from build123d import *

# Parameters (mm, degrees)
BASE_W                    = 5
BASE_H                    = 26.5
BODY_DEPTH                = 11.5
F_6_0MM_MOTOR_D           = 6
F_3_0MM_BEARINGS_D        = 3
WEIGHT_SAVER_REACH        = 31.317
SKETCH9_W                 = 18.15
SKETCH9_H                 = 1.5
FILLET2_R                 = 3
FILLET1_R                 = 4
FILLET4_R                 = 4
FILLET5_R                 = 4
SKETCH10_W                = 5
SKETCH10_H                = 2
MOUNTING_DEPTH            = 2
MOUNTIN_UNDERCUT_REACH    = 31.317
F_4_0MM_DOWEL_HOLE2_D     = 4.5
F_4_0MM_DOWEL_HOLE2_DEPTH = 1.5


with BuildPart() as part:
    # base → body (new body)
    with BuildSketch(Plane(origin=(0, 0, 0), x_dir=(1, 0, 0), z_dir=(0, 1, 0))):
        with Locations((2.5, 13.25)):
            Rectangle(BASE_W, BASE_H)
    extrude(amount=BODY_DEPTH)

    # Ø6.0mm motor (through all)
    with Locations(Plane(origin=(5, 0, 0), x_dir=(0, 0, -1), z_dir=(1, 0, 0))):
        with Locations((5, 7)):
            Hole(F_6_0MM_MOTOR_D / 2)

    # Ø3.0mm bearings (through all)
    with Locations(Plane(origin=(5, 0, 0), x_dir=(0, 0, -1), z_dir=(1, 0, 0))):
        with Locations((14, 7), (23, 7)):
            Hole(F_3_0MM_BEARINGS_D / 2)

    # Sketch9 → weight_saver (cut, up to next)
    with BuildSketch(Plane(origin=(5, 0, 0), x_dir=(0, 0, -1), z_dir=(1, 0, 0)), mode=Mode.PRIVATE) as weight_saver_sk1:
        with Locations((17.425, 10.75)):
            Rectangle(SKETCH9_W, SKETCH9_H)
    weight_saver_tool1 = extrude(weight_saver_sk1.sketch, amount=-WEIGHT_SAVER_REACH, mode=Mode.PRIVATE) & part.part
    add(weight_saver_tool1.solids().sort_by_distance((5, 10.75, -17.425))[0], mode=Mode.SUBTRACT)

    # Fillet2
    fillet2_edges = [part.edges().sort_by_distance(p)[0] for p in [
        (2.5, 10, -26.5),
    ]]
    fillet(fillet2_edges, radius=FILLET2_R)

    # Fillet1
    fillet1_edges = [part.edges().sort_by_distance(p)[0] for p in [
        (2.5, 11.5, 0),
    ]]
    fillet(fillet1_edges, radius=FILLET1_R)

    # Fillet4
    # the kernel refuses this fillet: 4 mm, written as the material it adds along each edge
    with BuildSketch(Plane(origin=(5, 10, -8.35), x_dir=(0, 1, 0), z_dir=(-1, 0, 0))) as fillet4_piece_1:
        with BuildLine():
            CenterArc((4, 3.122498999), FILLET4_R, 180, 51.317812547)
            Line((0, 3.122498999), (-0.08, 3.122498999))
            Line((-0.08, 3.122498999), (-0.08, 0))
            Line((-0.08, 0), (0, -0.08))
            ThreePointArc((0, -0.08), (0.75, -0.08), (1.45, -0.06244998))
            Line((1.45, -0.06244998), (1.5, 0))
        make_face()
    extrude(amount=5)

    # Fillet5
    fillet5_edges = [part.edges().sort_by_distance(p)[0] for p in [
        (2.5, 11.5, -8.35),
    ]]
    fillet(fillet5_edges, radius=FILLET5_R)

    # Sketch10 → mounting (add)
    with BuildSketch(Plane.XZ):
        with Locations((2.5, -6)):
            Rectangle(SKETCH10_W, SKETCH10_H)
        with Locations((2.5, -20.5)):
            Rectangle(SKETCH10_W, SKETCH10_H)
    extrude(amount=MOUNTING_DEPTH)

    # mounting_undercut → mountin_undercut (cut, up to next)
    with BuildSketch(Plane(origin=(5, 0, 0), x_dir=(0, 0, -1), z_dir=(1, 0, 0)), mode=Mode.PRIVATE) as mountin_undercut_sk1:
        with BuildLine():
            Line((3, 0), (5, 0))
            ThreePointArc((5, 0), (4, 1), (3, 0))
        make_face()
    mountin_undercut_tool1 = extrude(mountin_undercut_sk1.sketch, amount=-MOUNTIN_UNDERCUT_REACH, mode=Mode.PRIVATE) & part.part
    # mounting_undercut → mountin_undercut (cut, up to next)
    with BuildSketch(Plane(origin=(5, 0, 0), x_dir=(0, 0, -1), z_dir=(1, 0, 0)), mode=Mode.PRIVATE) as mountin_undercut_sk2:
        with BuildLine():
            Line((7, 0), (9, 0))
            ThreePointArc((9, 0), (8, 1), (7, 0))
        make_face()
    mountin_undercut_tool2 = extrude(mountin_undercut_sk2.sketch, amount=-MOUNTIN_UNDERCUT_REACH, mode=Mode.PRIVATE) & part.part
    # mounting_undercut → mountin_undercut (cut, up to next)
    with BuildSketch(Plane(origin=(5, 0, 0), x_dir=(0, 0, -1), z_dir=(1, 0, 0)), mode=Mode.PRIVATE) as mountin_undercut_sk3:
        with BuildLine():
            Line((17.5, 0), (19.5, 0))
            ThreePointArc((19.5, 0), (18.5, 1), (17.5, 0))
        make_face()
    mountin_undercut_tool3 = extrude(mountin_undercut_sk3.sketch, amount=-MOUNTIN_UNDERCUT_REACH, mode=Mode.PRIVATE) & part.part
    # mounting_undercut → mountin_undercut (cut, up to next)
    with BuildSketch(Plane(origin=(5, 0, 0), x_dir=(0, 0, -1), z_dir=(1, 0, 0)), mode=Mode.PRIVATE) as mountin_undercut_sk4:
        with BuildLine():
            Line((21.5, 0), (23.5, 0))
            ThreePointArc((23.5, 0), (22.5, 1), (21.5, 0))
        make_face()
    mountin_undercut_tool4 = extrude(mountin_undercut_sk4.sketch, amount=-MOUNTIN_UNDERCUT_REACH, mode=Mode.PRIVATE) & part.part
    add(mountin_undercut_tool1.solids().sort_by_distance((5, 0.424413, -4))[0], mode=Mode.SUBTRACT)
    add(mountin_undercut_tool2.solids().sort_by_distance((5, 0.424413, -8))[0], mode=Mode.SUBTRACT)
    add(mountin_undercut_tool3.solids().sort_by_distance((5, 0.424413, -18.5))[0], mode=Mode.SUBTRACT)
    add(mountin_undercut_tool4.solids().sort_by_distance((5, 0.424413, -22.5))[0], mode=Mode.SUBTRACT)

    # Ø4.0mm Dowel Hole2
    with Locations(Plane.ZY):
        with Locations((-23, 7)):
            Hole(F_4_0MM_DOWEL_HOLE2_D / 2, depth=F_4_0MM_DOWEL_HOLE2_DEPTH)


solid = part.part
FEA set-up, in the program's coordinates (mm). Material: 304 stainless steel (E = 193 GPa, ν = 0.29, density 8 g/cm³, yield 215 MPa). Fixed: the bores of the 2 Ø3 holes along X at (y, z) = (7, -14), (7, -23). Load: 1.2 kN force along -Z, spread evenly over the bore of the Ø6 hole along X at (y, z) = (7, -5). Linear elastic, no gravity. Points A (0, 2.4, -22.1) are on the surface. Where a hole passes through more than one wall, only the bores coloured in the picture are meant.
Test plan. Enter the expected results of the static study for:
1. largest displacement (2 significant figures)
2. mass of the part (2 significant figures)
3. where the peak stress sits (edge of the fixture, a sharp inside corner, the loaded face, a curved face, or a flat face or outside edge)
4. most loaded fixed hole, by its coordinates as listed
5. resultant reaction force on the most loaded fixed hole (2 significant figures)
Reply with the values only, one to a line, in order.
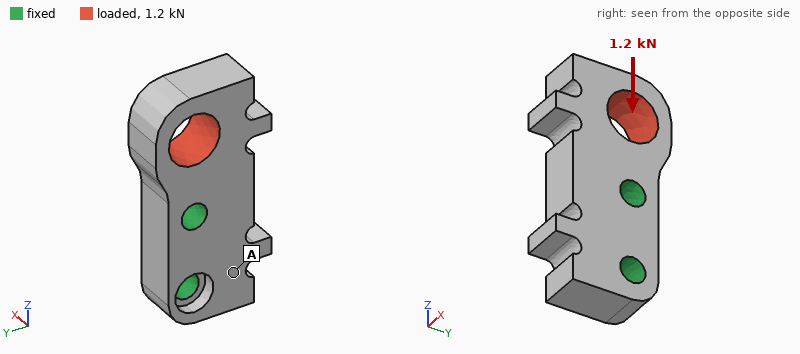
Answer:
5.8 µm
9.2 g
the loaded face
(7, -14)
1.1 kN
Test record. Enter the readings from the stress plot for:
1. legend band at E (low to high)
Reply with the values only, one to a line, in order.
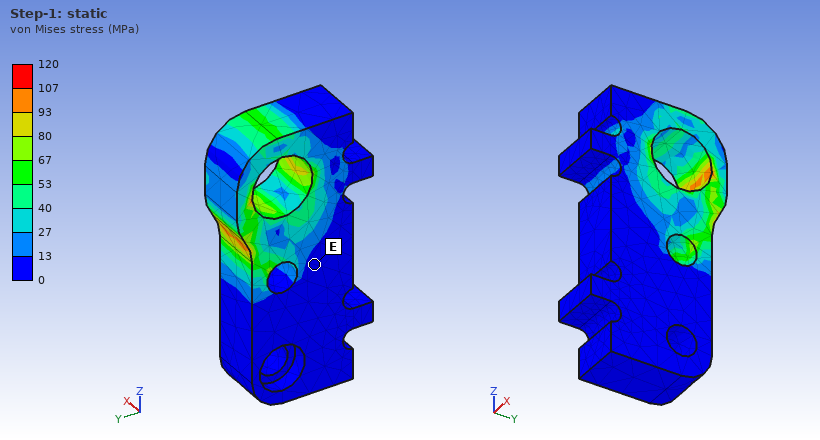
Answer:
0 to 13 MPa
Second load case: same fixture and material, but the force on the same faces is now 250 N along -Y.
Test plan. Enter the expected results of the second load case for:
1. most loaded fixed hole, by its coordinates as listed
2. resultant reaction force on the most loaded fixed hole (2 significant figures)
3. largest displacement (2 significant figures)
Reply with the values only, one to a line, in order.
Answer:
(7, -14)
380 N
5.4 µm
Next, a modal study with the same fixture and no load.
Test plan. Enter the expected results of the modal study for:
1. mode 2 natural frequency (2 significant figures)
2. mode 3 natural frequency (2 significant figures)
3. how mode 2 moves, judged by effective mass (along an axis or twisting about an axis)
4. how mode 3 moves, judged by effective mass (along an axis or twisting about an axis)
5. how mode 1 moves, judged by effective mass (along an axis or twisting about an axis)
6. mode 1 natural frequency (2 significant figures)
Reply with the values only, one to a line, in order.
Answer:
22 kHz
33 kHz
along Y
twisting about Z
along X
18 kHz
